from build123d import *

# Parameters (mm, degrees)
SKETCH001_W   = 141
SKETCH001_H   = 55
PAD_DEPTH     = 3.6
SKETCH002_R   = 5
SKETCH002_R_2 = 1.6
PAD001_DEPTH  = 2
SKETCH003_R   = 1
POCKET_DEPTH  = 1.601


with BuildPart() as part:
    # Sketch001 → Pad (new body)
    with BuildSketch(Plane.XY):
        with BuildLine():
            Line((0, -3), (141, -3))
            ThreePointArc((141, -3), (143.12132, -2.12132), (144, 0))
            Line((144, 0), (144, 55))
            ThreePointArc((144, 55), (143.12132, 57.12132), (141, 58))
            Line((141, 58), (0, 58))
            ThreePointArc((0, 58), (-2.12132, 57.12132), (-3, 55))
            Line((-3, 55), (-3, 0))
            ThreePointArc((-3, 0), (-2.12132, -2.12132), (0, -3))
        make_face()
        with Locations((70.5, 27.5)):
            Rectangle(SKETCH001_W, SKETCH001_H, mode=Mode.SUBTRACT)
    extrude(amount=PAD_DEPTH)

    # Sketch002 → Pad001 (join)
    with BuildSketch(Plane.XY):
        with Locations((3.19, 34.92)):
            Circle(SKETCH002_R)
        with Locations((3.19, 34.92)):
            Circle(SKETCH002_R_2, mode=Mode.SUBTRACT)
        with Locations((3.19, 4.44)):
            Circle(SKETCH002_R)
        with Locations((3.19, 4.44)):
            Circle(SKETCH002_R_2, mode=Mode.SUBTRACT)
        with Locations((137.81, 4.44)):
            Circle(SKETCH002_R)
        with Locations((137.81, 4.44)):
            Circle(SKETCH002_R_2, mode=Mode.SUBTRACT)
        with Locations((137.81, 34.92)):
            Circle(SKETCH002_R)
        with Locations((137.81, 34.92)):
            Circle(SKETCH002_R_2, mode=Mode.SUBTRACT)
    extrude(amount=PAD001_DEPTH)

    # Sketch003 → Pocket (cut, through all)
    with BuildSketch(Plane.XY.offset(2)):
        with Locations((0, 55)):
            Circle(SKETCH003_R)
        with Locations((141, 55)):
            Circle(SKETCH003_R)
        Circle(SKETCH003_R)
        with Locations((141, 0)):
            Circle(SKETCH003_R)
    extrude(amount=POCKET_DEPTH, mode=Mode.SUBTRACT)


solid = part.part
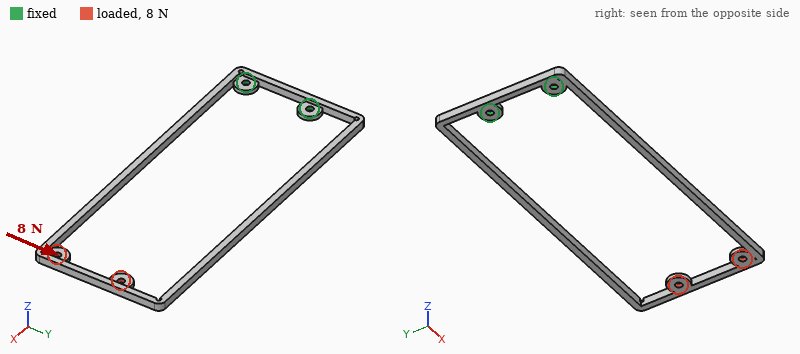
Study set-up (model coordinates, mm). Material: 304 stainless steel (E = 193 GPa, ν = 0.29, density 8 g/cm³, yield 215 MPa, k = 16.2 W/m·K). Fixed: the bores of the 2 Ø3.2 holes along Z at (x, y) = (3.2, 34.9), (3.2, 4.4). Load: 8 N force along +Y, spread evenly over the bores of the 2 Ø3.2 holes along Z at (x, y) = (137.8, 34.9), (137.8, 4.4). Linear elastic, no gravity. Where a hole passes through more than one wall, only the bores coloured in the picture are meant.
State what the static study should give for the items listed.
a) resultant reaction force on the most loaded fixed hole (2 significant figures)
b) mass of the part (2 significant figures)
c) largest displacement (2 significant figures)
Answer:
13 N
38 g
0.84 mm
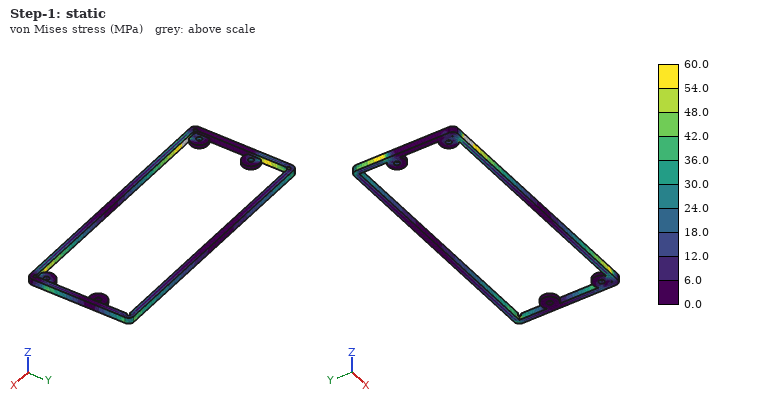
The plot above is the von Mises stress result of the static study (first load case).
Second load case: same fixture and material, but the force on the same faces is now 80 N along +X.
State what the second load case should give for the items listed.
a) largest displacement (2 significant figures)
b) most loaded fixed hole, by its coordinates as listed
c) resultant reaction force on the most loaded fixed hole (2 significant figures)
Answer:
0.30 mm
(3.2, 4.4)
62 N
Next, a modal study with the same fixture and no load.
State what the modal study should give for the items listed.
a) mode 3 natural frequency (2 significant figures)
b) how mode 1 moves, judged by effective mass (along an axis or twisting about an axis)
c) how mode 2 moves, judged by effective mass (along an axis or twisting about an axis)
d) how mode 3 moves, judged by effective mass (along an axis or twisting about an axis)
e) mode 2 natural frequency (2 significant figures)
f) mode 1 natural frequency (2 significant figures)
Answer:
250 Hz
along Z
along Y
twisting about X
120 Hz
82 Hz
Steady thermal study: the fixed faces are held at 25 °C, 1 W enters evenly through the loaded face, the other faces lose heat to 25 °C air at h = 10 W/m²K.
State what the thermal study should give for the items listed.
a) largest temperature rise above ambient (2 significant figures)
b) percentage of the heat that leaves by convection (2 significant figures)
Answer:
64 K
98 %
